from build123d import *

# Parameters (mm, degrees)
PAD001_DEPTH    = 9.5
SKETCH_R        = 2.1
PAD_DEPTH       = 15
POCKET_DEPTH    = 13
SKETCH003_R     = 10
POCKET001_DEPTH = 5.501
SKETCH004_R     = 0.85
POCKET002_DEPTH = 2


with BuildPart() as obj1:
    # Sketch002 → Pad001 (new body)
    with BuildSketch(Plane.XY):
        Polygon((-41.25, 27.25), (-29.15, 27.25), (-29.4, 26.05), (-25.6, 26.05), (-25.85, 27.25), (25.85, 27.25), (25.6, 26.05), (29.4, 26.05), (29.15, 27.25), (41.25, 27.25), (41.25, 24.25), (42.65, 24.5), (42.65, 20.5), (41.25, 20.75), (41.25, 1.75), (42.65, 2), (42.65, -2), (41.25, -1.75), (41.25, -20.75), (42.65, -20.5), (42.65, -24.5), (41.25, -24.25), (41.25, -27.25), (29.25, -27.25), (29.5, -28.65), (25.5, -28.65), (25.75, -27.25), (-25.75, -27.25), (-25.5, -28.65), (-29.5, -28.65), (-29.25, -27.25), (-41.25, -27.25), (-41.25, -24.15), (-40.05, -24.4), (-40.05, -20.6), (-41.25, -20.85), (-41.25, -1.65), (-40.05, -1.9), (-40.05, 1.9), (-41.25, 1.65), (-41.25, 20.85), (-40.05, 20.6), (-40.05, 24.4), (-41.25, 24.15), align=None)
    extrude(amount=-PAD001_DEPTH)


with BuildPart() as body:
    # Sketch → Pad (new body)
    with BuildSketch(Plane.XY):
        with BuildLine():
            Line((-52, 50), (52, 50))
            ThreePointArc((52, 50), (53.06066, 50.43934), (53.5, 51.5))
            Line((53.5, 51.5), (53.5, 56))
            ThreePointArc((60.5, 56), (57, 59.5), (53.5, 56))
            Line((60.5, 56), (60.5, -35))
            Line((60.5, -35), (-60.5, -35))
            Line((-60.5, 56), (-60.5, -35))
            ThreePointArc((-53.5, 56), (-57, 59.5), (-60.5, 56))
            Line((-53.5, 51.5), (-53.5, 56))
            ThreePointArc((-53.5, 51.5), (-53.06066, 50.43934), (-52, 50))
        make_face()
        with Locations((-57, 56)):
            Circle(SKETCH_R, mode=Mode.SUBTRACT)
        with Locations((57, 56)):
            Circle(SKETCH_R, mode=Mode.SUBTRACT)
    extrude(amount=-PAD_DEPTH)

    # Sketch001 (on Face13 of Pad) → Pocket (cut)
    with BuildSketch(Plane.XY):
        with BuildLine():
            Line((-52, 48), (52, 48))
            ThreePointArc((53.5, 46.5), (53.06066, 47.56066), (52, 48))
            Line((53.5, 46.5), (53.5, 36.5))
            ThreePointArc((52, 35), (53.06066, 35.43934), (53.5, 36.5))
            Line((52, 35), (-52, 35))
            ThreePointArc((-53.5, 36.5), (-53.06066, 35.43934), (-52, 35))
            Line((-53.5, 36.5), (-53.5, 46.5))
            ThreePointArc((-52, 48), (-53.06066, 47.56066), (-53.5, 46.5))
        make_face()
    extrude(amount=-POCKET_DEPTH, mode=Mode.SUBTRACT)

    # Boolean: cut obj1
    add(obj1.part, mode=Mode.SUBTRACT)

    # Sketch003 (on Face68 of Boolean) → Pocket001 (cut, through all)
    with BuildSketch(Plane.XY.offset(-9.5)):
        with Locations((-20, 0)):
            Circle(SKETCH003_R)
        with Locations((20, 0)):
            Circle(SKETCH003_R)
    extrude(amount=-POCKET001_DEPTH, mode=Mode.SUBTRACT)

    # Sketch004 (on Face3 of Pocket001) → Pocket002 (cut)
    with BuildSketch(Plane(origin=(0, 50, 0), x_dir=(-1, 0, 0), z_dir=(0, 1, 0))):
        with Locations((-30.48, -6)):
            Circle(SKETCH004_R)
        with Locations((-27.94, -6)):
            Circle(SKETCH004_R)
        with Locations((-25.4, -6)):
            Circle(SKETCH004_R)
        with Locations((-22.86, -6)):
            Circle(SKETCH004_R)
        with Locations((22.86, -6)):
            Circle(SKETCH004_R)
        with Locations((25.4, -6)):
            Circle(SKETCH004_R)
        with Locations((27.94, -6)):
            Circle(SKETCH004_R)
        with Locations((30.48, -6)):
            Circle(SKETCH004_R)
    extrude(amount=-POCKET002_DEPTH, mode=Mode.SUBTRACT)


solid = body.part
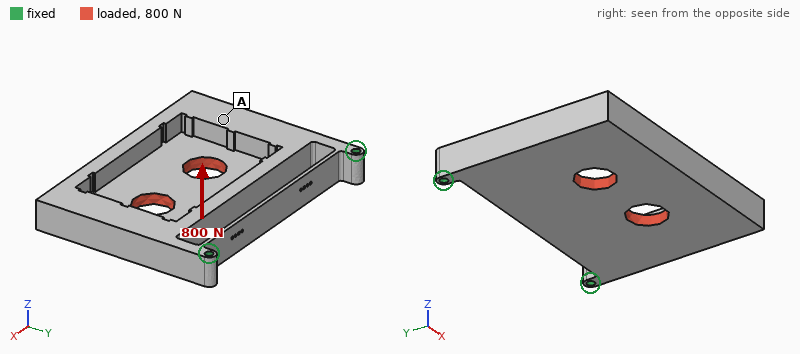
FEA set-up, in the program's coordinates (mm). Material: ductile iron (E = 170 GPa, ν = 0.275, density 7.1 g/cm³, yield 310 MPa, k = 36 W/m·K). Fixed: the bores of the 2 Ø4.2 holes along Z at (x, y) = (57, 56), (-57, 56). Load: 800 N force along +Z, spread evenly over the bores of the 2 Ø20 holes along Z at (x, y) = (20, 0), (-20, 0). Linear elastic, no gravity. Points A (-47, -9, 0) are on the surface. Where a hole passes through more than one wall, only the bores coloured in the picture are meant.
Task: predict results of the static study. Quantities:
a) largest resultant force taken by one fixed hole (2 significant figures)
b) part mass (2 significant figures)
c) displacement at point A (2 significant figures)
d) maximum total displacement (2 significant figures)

450 N
650 g
0.069 mm
0.11 mm
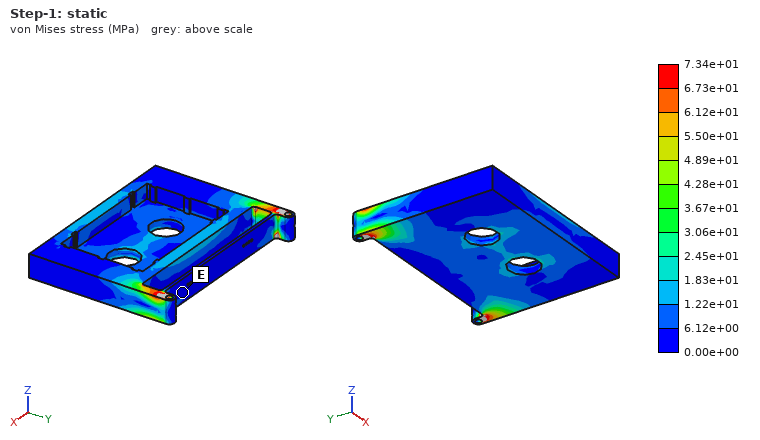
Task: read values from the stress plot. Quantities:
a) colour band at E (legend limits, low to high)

0.00e+00 to 6.12e+00 MPa
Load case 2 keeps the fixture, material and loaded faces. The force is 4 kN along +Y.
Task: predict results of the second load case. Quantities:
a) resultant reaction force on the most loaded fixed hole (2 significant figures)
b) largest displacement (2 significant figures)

2.1 kN
49 µm
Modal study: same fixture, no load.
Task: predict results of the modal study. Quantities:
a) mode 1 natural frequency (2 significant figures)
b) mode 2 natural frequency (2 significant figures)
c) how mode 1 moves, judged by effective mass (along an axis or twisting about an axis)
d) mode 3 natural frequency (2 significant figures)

690 Hz
1500 Hz
along Z
3000 Hz
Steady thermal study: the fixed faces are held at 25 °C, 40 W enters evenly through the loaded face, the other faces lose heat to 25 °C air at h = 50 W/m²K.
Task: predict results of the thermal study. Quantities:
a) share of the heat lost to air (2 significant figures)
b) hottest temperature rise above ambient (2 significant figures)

86 %
50 K
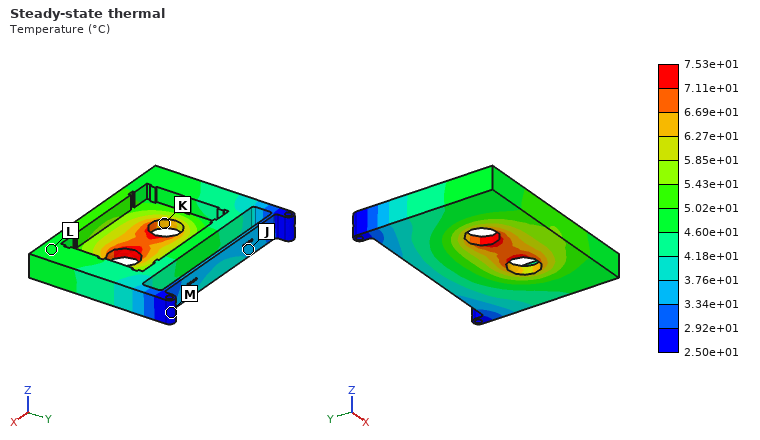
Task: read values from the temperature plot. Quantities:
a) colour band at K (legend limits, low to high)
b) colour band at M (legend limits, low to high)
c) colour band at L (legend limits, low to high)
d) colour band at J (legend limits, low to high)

6.27e+01 to 6.69e+01 °C
2.50e+01 to 2.92e+01 °C
4.60e+01 to 5.02e+01 °C
3.34e+01 to 3.76e+01 °C
